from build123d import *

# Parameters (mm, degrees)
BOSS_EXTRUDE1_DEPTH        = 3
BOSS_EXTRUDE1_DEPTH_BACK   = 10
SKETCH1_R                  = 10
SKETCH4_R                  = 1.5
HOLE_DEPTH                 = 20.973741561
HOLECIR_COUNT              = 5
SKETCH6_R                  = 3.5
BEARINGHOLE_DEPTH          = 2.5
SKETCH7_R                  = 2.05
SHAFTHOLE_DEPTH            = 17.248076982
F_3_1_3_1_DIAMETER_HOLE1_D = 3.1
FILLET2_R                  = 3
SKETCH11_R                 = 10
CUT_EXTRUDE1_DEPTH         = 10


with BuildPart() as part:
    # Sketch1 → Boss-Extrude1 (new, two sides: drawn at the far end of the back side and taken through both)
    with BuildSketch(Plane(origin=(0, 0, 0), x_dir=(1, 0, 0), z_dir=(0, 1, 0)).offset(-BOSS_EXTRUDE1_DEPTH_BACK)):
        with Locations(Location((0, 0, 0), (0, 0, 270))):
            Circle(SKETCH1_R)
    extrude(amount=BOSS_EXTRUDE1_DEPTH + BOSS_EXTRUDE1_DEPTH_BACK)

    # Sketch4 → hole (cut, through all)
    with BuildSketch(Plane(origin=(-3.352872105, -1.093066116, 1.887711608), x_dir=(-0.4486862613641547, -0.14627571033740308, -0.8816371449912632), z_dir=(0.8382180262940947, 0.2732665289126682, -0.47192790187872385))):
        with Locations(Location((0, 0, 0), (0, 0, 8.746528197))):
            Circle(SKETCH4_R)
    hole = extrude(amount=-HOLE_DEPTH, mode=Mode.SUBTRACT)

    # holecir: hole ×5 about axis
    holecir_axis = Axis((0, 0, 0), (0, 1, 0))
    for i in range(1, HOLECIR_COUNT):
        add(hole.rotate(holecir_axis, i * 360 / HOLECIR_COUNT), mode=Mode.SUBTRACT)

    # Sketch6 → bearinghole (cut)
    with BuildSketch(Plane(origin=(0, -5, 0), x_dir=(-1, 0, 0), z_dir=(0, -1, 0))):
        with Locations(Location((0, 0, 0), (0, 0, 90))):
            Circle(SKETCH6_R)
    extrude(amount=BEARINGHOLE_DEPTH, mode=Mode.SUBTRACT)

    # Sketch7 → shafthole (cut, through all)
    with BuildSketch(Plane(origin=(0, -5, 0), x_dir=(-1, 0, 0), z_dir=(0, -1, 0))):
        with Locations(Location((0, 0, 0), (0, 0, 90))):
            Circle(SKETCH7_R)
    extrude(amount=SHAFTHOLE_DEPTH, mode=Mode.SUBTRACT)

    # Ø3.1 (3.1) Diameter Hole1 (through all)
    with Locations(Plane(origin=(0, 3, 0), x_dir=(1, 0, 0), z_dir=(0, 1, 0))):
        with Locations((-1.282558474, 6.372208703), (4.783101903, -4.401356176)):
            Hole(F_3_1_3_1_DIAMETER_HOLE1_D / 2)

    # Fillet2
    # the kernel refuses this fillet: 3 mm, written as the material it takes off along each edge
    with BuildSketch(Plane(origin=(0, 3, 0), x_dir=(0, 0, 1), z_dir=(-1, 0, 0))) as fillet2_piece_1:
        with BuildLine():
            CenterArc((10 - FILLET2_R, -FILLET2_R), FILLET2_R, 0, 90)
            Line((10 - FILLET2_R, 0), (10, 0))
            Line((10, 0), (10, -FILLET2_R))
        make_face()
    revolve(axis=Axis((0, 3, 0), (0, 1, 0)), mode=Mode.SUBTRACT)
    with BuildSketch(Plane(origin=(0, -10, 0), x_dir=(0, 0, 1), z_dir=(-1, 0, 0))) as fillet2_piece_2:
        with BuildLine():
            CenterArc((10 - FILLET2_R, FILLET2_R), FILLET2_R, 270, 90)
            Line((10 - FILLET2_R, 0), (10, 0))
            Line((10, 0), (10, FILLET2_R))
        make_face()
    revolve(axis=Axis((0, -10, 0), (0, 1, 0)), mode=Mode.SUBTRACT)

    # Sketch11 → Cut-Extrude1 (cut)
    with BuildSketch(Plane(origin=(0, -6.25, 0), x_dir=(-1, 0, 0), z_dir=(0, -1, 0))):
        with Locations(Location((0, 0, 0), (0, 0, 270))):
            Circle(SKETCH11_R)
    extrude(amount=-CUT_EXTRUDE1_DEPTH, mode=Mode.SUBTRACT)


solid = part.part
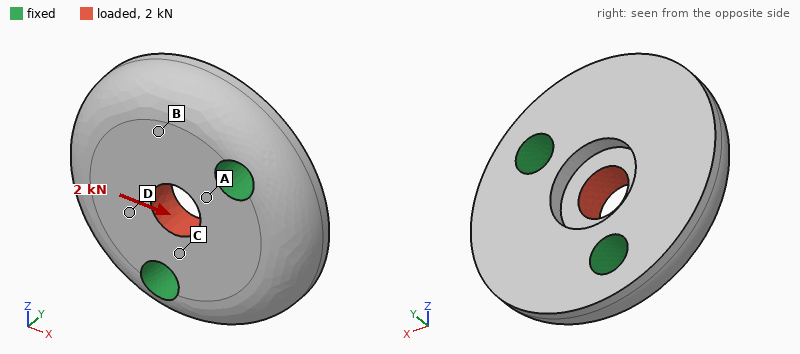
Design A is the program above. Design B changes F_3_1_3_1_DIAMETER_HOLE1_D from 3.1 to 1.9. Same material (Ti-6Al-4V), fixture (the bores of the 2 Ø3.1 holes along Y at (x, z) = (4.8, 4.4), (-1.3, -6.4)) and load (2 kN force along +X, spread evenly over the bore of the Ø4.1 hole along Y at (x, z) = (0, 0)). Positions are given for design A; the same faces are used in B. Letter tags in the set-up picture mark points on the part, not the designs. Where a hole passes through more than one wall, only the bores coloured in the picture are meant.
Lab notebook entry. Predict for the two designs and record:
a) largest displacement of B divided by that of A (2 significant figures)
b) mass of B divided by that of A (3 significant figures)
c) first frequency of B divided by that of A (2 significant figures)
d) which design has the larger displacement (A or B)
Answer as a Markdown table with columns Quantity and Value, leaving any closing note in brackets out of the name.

| Quantity | Value |
|---|---|
| largest displacement of B divided by that of A | 1.3 |
| mass of B divided by that of A | 1.04 |
| first frequency of B divided by that of A | 0.86 |
| which design has the larger displacement | B |
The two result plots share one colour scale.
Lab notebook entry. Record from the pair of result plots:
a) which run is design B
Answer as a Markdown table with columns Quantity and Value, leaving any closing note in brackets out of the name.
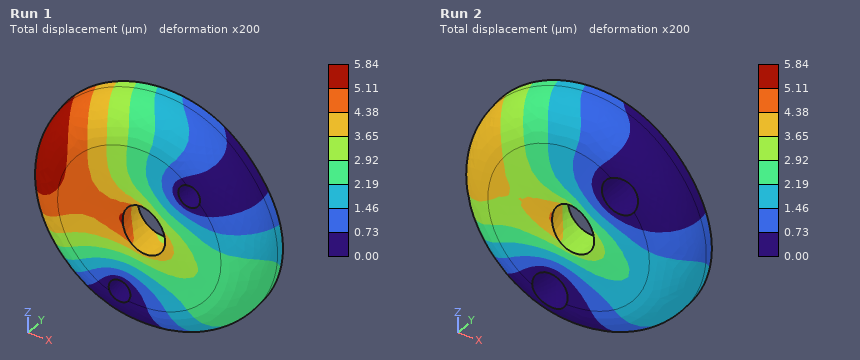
| Quantity | Value |
|---|---|
| which run is design B | Run 1 |
